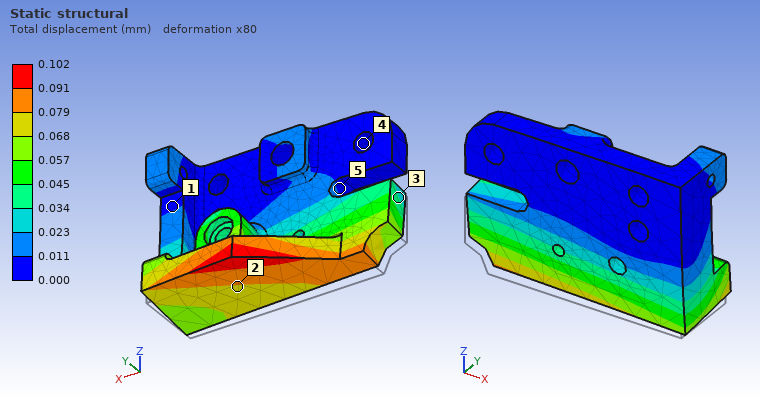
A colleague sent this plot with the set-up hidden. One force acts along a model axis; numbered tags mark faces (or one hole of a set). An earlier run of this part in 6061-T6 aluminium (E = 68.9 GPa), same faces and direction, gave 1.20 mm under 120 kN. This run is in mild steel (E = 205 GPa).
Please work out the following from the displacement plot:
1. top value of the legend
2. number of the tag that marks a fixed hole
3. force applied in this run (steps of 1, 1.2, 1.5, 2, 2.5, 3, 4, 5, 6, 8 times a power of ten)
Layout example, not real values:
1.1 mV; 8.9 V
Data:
0.102 mm; 4; 30 kN
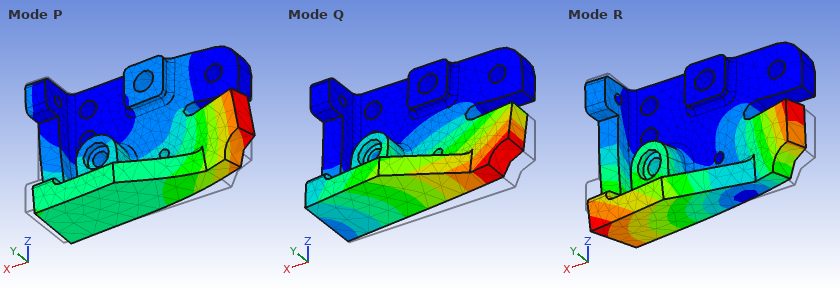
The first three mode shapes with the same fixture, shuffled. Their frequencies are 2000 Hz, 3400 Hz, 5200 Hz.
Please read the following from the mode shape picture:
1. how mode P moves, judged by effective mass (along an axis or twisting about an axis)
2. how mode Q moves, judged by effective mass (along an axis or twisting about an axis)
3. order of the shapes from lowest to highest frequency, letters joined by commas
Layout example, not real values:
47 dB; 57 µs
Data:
along X; along Y; Q, R, P
